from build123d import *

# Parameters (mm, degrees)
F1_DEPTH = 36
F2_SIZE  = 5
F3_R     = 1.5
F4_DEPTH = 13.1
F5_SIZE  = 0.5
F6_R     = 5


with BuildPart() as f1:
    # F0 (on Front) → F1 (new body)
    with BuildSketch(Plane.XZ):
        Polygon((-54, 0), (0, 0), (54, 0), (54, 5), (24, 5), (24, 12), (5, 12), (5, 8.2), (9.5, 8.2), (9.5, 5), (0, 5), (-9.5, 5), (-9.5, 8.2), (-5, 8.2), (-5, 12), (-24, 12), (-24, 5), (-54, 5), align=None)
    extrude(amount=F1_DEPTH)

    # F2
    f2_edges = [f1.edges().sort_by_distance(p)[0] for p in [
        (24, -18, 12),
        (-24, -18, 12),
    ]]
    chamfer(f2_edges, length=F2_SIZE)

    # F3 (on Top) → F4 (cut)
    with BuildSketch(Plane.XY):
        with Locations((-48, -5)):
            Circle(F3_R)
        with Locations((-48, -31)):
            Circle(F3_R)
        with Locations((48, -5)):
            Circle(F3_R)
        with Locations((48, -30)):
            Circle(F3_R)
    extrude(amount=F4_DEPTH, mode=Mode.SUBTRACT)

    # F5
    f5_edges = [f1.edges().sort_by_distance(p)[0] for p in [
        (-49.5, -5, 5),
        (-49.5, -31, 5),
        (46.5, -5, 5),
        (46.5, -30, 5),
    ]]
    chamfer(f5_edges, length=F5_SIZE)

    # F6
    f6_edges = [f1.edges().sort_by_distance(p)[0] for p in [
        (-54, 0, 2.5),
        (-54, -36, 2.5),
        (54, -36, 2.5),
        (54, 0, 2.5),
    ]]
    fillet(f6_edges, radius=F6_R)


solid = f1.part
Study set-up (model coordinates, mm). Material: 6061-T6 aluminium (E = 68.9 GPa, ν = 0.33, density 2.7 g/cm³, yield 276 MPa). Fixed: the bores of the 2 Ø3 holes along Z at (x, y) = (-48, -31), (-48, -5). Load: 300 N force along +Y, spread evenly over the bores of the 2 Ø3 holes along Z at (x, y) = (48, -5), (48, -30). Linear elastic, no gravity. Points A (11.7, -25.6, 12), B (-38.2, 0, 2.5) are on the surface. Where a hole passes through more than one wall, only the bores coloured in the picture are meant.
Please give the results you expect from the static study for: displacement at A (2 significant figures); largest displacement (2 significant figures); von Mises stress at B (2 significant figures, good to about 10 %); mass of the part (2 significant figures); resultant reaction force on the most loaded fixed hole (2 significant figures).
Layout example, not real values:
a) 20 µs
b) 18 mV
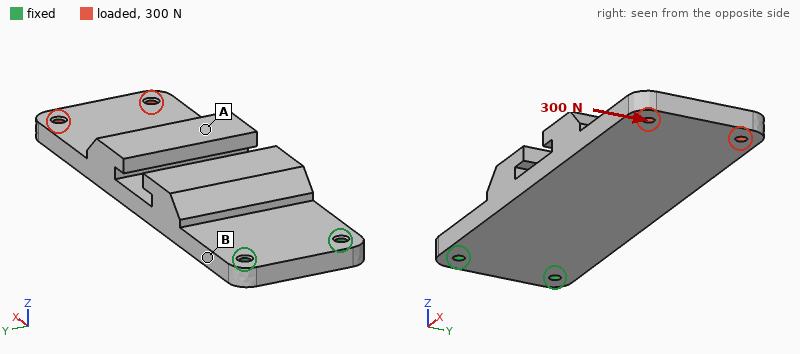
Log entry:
a) 34 µm
b) 82 µm
c) 23 MPa
d) 72 g
e) 1.1 kN
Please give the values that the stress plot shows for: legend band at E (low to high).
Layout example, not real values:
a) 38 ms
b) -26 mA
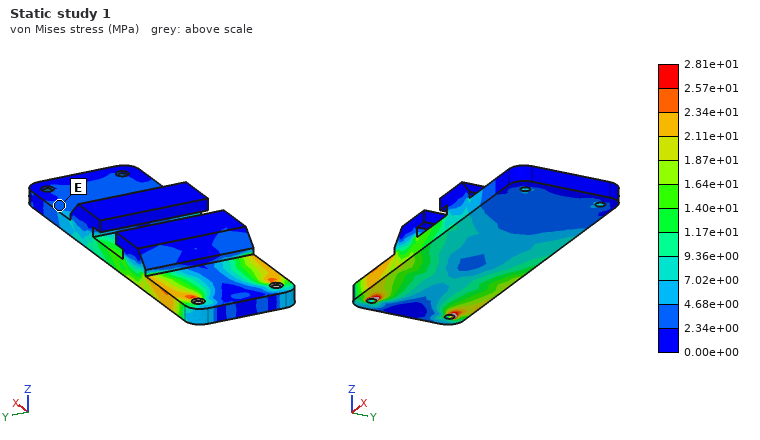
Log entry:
a) 2.34e+00 to 4.68e+00 MPa
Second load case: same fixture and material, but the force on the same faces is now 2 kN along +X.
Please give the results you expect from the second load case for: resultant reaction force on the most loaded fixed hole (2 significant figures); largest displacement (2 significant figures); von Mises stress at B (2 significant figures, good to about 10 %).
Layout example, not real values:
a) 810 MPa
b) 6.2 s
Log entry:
a) 1.0 kN
b) 0.12 mm
c) 15 MPa
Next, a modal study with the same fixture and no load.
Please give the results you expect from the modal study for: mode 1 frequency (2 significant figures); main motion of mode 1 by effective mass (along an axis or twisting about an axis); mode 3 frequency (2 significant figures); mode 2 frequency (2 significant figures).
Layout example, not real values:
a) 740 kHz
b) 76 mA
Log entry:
a) 370 Hz
b) along Z
c) 2300 Hz
d) 2200 Hz
